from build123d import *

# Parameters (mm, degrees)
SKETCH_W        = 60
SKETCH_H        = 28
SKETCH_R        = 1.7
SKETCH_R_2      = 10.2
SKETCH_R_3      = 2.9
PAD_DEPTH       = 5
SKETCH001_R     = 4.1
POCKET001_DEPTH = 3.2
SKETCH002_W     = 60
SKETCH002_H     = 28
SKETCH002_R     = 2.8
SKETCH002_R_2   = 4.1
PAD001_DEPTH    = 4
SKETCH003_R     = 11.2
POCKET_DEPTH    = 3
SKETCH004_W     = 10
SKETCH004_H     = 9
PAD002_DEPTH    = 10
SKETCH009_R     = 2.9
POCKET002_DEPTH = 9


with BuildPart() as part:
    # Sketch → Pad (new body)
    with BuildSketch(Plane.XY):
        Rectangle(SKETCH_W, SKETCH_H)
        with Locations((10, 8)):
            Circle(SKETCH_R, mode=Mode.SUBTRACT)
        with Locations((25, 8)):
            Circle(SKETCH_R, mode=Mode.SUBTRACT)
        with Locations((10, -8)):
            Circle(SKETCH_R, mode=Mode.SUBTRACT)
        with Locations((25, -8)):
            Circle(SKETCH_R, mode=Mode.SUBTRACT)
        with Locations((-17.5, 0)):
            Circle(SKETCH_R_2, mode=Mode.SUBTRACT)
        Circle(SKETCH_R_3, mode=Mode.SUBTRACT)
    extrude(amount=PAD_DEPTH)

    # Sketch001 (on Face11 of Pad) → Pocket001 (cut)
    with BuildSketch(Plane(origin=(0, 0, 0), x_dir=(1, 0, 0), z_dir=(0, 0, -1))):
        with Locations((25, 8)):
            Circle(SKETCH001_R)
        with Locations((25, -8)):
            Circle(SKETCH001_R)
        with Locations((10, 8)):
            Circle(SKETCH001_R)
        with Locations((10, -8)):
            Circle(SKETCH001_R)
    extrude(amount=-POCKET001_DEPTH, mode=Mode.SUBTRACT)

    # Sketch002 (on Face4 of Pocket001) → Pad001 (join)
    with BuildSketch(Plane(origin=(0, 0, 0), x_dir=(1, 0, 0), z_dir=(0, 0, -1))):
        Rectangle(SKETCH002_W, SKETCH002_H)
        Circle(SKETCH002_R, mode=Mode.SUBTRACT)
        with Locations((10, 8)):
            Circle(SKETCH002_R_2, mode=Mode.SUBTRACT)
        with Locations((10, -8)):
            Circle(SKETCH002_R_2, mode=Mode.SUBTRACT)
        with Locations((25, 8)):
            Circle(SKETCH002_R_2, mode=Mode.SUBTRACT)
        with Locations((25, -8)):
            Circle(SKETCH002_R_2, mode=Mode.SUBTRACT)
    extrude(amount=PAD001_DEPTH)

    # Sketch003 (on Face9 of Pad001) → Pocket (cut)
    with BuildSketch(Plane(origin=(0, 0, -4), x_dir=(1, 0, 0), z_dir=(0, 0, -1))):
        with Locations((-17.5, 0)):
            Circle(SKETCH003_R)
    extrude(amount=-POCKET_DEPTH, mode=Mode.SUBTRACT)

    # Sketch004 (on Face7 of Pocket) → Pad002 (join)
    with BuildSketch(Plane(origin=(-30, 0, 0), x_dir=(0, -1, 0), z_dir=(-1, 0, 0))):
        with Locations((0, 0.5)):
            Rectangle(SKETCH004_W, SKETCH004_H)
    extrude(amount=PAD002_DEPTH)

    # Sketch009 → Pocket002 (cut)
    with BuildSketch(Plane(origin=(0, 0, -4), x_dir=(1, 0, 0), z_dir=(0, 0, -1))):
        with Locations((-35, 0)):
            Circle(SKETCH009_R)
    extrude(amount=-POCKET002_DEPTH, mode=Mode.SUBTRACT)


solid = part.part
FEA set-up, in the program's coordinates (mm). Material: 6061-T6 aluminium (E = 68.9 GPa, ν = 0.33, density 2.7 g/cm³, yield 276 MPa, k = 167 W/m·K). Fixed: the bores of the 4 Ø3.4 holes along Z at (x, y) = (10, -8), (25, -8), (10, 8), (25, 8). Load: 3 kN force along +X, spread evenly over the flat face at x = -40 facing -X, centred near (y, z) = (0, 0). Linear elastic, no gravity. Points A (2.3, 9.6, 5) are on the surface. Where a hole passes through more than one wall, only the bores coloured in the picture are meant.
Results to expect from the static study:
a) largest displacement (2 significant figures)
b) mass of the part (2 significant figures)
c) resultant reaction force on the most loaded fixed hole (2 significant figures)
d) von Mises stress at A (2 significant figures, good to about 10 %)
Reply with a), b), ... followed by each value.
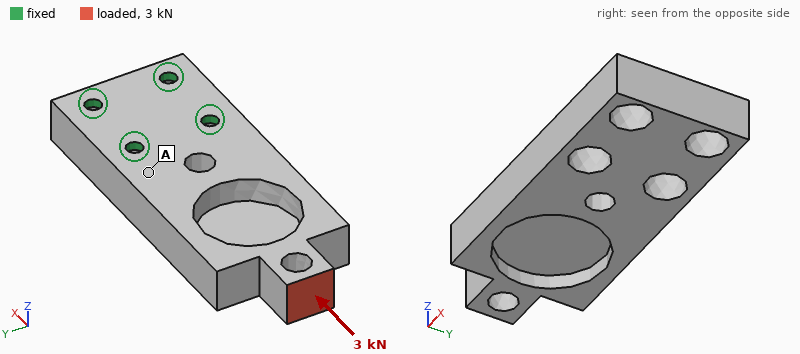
a) 68 µm
b) 30 g
c) 1.0 kN
d) 23 MPa
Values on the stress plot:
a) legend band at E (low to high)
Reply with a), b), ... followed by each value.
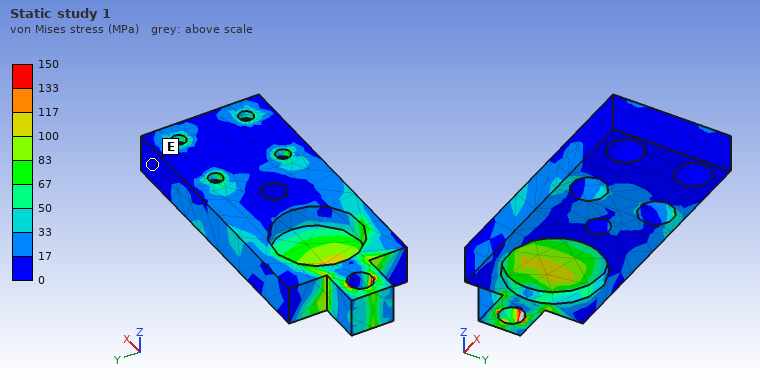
a) 0 to 17 MPa
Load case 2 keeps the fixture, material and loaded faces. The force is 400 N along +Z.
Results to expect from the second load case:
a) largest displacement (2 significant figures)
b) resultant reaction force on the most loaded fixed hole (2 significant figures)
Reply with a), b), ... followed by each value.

a) 0.42 mm
b) 970 N
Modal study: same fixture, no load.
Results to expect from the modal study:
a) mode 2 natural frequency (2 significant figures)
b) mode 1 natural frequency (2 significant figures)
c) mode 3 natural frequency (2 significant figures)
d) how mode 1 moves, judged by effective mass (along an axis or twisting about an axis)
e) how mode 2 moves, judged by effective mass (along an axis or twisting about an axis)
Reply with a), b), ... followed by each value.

a) 6700 Hz
b) 2800 Hz
c) 8000 Hz
d) along Z
e) along Y
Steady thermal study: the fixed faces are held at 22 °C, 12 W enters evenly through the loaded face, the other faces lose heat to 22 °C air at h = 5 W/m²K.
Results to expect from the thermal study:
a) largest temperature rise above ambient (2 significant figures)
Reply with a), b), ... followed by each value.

a) 42 K
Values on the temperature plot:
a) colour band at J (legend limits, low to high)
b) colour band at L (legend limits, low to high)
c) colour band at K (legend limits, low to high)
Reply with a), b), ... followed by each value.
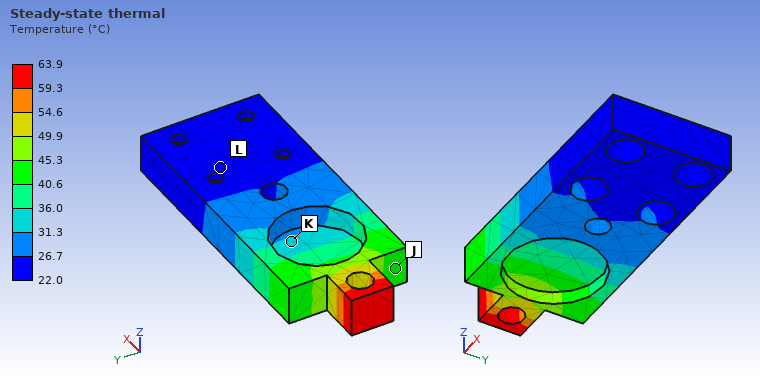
a) 40.6 to 45.3 °C
b) 22.0 to 26.7 °C
c) 31.3 to 36.0 °C
